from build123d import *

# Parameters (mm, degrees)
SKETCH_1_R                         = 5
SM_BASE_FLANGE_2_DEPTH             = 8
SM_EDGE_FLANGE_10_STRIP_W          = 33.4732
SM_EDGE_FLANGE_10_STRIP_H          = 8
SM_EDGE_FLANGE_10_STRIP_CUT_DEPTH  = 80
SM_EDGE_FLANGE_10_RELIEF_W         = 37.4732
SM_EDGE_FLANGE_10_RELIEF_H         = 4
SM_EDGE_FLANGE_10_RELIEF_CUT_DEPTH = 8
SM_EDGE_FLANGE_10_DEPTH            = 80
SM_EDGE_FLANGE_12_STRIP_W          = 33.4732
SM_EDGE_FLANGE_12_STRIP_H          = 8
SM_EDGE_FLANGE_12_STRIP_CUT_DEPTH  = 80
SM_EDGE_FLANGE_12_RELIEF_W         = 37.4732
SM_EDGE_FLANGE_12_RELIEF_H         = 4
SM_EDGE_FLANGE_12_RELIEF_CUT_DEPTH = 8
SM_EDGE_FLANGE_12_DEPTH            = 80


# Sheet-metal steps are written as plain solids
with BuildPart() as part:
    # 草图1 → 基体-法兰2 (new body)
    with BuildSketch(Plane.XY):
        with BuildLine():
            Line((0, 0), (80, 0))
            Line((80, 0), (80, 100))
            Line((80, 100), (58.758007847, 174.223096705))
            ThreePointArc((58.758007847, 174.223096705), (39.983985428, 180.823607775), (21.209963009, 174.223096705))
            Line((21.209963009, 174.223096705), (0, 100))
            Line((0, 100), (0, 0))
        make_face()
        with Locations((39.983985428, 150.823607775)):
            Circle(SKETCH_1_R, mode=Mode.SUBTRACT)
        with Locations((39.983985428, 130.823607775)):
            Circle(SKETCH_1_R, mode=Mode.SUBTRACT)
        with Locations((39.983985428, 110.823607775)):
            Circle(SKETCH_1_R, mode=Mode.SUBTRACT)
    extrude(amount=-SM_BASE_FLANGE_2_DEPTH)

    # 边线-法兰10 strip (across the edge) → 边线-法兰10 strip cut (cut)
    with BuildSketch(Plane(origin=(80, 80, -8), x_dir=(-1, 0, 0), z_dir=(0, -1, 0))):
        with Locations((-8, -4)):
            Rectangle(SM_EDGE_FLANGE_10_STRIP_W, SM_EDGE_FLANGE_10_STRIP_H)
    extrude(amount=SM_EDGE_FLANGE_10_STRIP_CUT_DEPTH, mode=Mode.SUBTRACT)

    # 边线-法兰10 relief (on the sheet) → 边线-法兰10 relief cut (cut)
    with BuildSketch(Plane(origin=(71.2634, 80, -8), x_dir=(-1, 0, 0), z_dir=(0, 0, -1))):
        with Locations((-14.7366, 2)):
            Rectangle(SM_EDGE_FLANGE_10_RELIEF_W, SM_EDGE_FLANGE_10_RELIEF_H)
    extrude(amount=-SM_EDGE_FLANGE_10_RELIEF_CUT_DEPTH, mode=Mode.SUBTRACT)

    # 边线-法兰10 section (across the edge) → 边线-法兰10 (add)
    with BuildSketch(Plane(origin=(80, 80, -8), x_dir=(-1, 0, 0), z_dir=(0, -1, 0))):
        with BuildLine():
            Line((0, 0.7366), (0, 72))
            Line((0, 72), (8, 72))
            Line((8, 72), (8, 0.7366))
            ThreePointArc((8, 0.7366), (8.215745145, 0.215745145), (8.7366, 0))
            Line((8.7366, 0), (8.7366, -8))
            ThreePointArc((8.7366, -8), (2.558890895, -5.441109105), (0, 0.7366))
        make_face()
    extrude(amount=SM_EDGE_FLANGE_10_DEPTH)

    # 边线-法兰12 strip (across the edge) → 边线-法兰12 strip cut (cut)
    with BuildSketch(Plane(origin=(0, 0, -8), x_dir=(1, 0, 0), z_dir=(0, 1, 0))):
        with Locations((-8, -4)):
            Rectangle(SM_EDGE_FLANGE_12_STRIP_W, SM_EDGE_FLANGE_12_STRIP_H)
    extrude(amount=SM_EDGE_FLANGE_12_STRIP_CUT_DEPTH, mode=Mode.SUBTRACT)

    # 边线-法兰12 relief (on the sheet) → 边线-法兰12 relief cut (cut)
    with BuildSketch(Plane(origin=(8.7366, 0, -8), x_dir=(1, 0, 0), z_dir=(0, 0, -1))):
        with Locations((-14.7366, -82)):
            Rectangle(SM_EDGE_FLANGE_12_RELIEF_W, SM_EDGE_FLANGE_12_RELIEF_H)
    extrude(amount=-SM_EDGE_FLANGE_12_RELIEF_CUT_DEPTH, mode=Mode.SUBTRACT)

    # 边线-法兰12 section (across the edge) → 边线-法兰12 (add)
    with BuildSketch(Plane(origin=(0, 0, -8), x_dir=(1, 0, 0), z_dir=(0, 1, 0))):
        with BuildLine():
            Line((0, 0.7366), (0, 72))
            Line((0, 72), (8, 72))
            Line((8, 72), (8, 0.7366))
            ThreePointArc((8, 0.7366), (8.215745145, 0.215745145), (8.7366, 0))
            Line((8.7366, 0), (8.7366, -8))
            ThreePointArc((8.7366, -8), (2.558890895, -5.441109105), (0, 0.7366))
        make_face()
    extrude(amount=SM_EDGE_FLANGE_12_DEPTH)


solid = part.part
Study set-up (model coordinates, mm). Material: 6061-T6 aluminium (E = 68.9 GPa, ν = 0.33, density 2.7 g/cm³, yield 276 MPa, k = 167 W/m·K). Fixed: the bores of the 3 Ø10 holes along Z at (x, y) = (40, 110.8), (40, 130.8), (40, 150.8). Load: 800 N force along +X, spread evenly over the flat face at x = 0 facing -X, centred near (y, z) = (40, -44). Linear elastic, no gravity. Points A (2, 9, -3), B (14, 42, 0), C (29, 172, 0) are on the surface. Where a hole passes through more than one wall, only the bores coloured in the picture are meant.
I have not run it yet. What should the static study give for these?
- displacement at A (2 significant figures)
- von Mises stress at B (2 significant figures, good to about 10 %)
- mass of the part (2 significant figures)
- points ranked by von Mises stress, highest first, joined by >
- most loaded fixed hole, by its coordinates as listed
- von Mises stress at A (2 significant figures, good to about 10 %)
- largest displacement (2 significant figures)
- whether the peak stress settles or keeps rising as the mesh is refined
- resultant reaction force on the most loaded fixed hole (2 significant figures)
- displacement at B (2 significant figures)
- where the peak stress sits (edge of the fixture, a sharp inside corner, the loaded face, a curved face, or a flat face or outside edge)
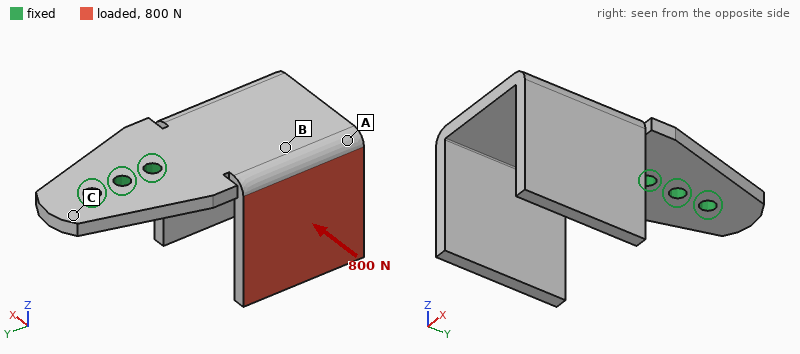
0.28 mm
33 MPa
510 g
B > A > C
(40, 110.8)
15 MPa
0.96 mm
keeps rising
1.9 kN
0.15 mm
a sharp inside corner
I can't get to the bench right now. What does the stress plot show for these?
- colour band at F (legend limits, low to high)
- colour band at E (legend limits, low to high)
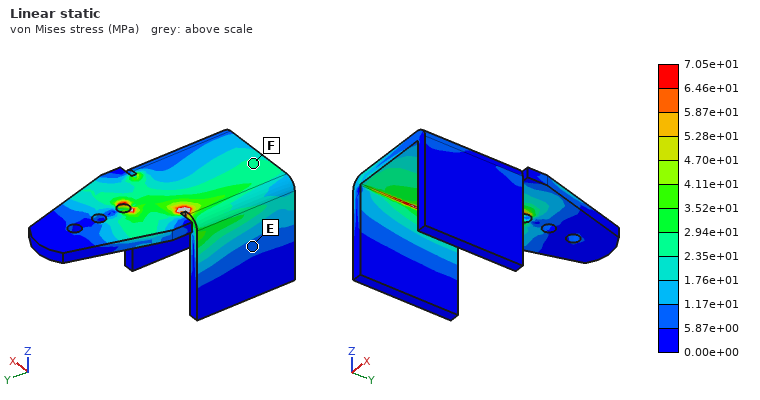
2.35e+01 to 2.94e+01 MPa
5.87e+00 to 1.17e+01 MPa
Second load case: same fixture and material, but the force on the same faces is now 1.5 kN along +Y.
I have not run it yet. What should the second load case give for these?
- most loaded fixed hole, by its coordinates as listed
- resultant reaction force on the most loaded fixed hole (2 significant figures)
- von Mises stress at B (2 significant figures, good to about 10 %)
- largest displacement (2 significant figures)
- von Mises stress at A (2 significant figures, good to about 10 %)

(40, 110.8)
2.0 kN
20 MPa
2.0 mm
14 MPa
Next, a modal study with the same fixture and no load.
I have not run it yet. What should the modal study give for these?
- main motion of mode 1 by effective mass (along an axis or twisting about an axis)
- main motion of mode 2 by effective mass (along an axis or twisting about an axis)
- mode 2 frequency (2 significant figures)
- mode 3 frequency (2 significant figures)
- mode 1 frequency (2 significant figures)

along Z
along X
360 Hz
710 Hz
250 Hz
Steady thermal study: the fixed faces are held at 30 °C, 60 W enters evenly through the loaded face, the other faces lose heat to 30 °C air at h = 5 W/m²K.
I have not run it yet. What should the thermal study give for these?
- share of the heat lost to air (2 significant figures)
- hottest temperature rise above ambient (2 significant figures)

12 %
69 K
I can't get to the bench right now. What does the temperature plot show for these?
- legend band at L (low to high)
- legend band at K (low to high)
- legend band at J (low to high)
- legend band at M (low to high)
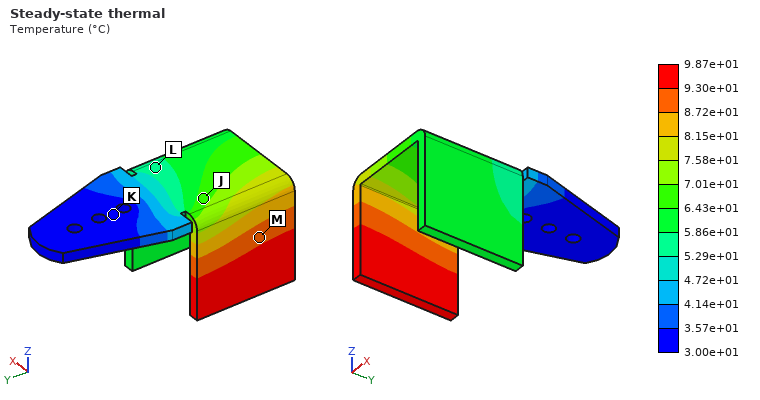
5.29e+01 to 5.86e+01 °C
3.00e+01 to 3.57e+01 °C
6.43e+01 to 7.01e+01 °C
8.72e+01 to 9.30e+01 °C
